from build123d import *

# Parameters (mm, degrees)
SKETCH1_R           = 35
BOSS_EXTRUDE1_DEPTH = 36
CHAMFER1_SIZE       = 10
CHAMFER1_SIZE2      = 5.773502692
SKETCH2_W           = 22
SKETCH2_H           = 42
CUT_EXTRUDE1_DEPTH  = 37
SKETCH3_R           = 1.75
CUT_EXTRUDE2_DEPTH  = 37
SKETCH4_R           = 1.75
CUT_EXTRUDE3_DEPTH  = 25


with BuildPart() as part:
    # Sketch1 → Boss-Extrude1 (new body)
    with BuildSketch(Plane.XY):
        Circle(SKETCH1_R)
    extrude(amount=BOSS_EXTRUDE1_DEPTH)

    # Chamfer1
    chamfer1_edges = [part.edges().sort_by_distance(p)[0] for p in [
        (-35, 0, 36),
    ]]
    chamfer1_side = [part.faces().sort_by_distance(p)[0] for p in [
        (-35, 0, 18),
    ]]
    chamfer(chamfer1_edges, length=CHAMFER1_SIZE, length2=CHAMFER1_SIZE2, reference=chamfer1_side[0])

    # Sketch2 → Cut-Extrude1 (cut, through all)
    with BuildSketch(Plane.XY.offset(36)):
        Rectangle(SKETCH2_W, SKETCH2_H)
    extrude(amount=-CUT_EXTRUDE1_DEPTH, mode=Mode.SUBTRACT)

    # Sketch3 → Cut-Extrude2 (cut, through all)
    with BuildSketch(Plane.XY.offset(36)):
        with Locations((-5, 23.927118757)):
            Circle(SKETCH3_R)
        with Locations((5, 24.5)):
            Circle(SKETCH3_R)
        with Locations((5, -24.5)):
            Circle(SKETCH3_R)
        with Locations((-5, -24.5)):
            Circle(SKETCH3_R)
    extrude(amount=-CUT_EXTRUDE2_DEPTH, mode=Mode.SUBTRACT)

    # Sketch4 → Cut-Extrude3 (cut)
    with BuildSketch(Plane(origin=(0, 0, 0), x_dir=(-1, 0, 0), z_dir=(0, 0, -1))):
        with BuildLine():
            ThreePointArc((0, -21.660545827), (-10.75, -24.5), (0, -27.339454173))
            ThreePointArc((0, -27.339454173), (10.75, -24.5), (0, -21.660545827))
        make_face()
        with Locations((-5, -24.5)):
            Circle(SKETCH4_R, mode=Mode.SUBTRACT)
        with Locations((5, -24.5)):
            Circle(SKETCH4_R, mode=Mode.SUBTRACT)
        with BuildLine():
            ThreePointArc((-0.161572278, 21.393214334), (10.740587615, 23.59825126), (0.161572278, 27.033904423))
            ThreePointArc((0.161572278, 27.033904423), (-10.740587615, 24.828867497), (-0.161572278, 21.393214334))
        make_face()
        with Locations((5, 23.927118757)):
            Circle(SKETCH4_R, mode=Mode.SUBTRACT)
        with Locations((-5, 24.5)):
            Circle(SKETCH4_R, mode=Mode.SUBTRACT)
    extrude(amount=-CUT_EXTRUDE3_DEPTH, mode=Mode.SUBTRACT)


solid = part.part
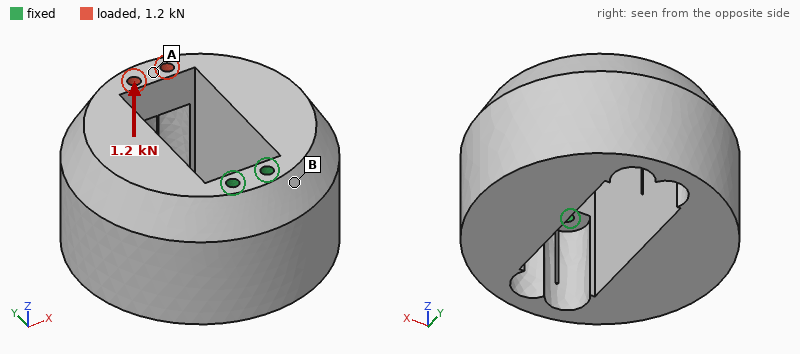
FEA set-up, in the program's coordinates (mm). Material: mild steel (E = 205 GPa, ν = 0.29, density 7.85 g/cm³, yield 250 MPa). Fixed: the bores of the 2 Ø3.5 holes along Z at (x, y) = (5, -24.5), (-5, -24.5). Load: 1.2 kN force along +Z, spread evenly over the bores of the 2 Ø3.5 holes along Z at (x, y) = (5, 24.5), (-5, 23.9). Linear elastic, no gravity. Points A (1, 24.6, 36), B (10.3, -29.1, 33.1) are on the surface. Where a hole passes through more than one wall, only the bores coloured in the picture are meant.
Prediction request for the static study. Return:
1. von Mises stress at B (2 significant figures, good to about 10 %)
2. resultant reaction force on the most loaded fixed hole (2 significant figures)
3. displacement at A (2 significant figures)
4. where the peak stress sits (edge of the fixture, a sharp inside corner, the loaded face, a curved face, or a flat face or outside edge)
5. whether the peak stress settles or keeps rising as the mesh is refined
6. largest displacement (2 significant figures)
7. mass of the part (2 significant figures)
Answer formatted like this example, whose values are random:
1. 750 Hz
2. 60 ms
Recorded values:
1. 81 MPa
2. 780 N
3. 73 µm
4. edge of the fixture
5. keeps rising
6. 95 µm
7. 710 g
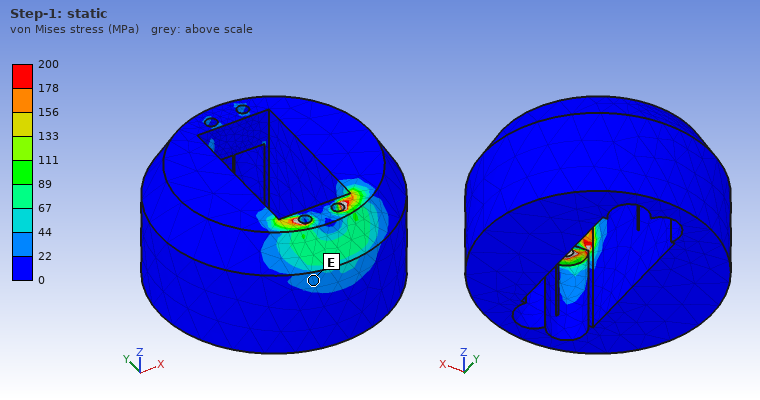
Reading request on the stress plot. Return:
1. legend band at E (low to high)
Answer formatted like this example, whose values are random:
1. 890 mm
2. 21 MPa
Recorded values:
1. 22 to 44 MPa
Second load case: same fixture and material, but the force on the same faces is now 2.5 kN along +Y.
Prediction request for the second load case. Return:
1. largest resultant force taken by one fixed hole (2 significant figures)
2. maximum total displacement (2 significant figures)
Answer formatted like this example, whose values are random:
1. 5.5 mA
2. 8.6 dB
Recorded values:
1. 1.4 kN
2. 11 µm
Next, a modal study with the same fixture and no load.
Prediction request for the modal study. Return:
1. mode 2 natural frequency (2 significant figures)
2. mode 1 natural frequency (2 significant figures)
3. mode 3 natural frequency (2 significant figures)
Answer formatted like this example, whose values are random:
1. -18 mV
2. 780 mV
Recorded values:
1. 460 Hz
2. 410 Hz
3. 700 Hz
